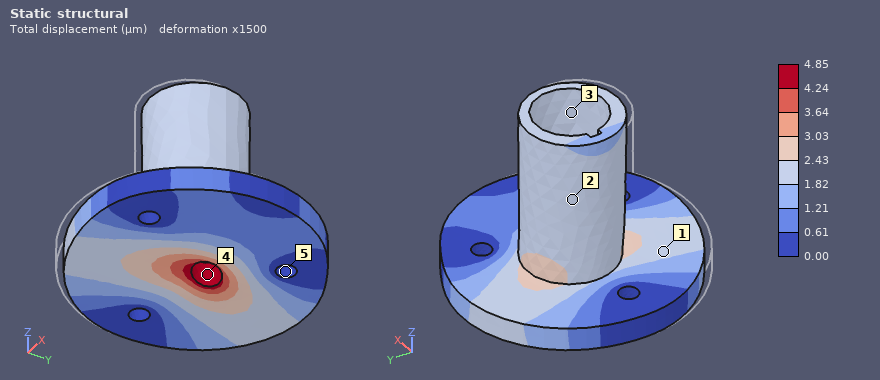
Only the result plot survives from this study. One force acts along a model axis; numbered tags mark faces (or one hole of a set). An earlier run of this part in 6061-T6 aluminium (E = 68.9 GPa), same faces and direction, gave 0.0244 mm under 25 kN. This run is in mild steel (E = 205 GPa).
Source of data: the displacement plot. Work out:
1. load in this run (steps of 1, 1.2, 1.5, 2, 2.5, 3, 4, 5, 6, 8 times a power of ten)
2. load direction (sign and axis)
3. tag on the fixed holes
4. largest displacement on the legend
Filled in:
15 kN
+Y
5
4.85 µm
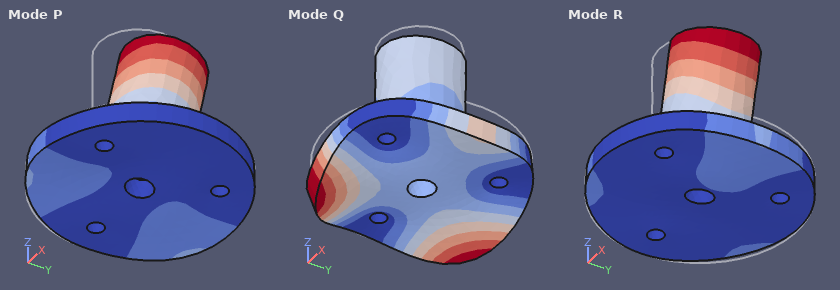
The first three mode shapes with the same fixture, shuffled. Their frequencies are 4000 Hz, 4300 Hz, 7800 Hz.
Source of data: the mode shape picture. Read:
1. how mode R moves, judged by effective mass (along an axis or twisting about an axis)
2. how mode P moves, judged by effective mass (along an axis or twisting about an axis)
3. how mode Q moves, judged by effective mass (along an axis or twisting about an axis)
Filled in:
along X
along Y
along Z
